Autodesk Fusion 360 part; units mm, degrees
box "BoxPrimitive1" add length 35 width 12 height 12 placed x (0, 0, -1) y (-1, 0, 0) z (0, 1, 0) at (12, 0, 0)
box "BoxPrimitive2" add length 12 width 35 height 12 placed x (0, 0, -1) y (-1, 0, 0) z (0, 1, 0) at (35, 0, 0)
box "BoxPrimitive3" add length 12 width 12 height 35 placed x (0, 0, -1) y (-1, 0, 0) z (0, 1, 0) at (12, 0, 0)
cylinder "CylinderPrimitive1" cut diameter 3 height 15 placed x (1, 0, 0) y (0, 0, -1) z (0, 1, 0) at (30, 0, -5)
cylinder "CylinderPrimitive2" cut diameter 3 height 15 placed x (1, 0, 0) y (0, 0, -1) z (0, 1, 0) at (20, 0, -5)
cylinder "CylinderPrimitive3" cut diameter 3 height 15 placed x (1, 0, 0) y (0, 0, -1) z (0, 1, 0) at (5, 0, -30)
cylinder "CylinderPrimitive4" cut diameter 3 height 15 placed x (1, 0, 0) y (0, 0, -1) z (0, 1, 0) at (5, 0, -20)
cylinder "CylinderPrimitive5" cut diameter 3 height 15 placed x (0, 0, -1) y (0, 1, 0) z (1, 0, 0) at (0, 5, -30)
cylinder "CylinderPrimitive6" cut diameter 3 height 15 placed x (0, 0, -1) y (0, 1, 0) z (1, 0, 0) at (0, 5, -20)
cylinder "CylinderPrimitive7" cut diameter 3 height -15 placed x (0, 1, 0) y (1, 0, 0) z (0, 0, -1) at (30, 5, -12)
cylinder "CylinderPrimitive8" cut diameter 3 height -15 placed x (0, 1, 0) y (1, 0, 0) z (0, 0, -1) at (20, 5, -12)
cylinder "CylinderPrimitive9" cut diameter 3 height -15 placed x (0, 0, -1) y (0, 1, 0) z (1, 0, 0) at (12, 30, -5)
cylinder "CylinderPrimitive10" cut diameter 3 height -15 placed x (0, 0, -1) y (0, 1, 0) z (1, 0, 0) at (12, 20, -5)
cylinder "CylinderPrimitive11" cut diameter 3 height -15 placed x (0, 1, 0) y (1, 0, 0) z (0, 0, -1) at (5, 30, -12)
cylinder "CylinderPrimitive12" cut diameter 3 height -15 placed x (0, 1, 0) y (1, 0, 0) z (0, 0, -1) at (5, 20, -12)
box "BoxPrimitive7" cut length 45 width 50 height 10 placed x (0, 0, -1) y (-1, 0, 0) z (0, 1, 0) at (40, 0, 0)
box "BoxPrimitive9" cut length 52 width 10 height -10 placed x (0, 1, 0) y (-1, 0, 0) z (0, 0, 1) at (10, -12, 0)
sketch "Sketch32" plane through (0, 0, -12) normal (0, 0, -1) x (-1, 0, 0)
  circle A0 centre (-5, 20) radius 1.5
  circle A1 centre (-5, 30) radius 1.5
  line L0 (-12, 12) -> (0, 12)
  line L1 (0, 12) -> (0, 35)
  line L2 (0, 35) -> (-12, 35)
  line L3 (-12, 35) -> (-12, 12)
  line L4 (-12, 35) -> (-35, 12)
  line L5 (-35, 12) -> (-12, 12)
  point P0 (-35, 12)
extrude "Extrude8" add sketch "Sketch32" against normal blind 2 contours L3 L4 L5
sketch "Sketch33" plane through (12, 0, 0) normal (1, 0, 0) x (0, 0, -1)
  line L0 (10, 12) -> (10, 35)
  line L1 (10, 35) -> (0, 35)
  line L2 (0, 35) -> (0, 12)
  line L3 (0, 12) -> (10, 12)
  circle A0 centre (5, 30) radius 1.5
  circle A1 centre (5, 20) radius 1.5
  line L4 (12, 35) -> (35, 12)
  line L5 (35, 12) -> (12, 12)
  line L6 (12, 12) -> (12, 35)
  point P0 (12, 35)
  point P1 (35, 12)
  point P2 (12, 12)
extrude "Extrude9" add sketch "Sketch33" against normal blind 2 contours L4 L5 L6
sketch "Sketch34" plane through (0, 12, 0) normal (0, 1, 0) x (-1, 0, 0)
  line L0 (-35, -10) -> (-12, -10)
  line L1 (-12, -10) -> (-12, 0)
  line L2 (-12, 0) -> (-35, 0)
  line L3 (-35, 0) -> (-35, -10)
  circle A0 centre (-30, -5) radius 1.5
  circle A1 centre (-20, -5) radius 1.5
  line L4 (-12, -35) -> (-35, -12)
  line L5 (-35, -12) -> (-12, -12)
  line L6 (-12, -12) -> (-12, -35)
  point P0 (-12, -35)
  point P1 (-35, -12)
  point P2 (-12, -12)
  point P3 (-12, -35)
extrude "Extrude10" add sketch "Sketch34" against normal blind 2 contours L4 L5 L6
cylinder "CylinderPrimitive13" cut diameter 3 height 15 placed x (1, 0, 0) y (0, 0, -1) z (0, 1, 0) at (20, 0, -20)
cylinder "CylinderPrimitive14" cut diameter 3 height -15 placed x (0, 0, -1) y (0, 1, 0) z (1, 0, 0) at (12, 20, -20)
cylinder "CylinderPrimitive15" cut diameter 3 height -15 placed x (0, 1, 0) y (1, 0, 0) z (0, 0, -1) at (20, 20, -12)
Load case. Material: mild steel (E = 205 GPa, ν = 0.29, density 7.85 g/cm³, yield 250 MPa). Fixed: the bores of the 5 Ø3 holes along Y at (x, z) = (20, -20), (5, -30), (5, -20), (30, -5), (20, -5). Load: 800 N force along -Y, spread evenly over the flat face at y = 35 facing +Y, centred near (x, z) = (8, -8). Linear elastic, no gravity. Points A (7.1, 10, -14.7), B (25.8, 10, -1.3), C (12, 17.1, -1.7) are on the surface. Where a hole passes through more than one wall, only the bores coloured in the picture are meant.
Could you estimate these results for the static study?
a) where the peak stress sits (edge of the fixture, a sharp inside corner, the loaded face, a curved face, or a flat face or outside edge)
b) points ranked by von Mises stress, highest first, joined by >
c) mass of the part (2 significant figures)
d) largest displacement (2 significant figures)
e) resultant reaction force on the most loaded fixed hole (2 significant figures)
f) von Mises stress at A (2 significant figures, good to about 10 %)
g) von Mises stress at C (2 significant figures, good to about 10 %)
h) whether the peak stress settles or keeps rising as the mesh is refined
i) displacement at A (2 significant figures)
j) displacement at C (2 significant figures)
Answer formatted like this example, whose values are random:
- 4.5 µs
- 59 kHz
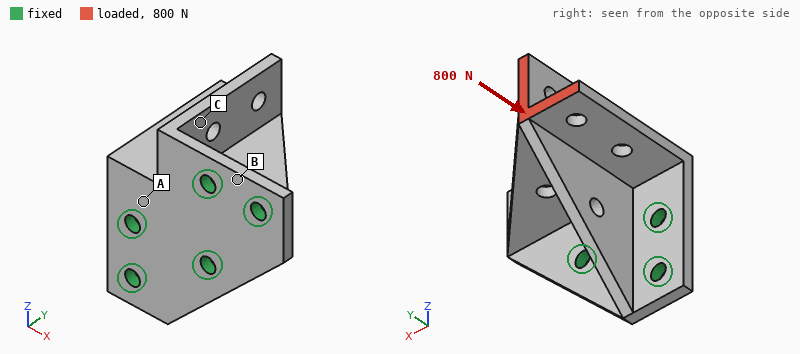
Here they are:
- edge of the fixture
- A > C > B
- 29 g
- 39 µm
- 550 N
- 73 MPa
- 41 MPa
- keeps rising
- 8.1 µm
- 22 µm
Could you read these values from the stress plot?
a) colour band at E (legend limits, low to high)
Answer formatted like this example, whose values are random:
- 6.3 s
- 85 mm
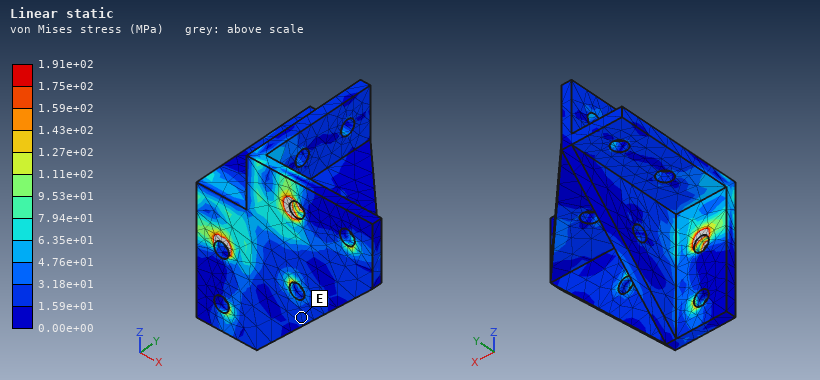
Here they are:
- 1.59e+01 to 3.18e+01 MPa
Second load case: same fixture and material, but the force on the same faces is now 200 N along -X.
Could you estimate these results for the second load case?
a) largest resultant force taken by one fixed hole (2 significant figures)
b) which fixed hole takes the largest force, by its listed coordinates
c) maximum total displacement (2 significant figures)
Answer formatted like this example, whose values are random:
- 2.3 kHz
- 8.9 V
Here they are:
- 210 N
- (5, -20)
- 38 µm
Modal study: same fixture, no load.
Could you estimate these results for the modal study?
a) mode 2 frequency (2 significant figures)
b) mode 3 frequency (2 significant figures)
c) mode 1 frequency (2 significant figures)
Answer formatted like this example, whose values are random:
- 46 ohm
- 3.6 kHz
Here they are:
- 8700 Hz
- 14 kHz
- 6800 Hz
